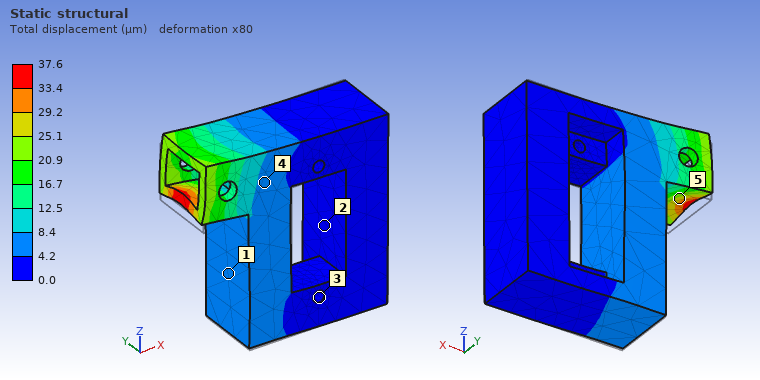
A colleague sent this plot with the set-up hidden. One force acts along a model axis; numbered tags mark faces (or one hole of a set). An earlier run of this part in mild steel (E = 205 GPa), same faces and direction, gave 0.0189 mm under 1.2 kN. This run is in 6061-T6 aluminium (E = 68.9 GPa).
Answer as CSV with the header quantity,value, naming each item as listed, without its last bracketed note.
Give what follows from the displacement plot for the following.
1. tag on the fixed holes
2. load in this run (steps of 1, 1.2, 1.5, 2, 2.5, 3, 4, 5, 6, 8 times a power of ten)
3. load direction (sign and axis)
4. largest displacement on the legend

quantity,value
tag on the fixed holes,3
load in this run,800 N
load direction,+Z
largest displacement on the legend,37.6 µm
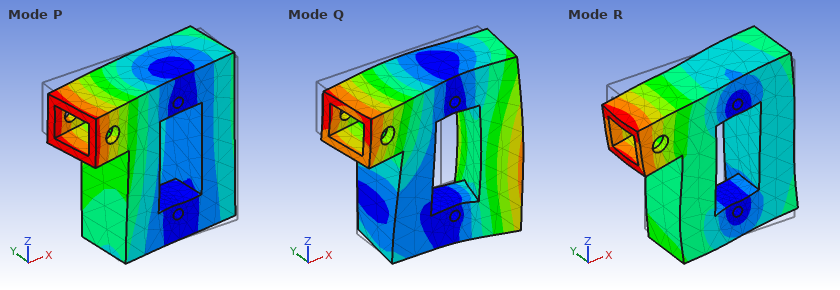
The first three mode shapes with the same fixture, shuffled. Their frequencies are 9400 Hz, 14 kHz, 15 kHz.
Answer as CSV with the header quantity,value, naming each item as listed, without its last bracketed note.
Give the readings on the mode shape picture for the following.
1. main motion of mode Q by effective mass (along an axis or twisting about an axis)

quantity,value
main motion of mode Q by effective mass,along Y
